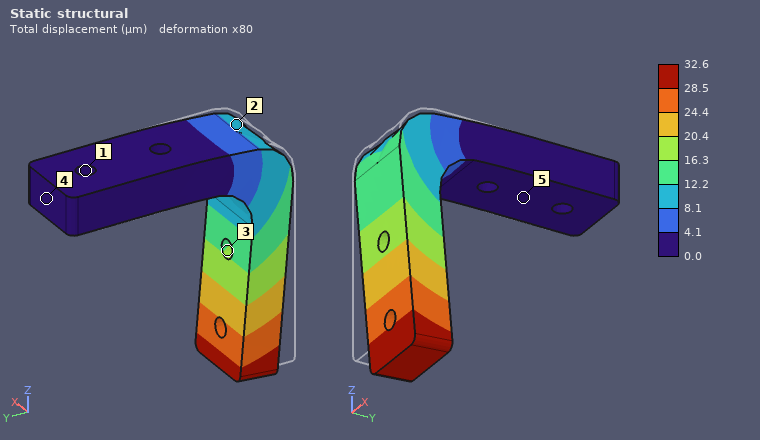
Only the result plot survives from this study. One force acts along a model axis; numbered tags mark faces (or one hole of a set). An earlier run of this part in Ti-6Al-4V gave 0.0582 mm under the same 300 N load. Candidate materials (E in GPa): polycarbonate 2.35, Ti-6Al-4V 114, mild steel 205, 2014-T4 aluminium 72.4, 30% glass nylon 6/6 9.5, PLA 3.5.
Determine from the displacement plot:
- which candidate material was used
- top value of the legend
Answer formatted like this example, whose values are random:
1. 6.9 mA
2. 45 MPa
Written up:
1. mild steel
2. 32.6 µm
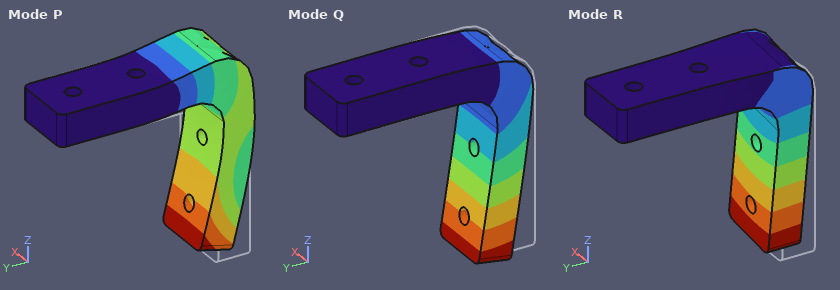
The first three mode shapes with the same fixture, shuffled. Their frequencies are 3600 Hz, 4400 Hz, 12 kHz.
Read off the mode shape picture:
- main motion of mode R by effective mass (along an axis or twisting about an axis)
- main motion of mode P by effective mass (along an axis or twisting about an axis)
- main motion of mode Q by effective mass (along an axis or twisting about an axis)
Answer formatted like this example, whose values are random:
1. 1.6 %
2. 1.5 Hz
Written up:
1. along X
2. along Z
3. along Y
